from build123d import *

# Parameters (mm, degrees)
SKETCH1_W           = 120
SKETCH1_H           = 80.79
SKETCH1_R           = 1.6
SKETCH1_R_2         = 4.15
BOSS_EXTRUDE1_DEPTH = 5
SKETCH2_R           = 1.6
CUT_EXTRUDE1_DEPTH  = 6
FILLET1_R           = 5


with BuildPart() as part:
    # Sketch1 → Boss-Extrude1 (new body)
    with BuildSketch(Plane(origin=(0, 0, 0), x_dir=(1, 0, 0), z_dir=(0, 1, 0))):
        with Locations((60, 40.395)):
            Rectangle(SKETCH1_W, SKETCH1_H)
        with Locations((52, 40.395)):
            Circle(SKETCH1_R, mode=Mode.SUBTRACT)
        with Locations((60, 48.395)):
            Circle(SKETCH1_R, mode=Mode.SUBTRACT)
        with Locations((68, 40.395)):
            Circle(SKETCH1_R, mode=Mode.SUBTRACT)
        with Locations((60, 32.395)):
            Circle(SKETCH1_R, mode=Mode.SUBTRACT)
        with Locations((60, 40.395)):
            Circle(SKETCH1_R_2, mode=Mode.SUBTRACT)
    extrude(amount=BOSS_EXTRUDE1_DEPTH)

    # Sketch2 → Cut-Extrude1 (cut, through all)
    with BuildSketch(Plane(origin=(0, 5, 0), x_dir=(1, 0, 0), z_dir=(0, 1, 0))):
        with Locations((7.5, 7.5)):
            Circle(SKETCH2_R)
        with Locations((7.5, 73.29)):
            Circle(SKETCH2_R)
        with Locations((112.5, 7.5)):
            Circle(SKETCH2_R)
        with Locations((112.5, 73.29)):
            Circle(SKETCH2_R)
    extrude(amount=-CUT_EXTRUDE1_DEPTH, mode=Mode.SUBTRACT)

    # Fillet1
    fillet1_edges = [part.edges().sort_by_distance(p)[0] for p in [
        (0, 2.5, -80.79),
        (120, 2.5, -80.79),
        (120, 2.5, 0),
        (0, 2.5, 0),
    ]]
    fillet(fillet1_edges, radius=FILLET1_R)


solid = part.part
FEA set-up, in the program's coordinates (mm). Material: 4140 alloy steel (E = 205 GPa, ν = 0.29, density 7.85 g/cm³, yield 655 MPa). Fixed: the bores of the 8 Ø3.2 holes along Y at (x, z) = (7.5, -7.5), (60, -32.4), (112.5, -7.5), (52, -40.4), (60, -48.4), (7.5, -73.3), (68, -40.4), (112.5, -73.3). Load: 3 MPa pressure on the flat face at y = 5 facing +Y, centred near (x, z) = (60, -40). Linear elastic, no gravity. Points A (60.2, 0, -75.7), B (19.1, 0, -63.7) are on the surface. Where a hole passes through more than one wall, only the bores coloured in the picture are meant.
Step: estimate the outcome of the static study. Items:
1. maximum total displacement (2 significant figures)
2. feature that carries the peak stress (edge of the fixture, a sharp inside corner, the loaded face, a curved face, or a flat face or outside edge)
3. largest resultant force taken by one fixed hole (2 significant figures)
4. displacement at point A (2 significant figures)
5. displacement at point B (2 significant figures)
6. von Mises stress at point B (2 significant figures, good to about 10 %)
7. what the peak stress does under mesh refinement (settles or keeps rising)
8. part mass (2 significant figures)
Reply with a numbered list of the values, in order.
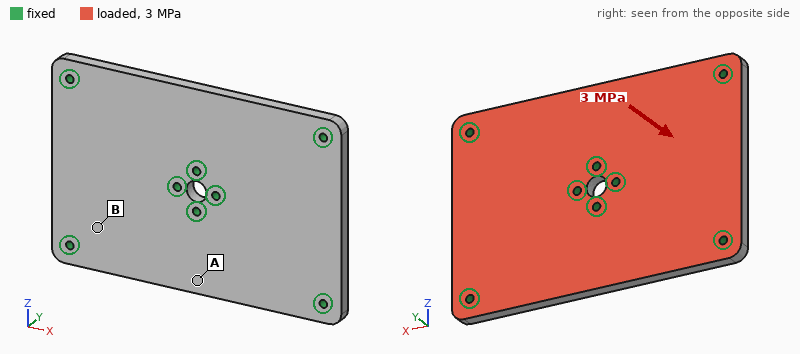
1. 0.15 mm
2. edge of the fixture
3. 4.0 kN
4. 0.12 mm
5. 0.044 mm
6. 130 MPa
7. keeps rising
8. 380 g
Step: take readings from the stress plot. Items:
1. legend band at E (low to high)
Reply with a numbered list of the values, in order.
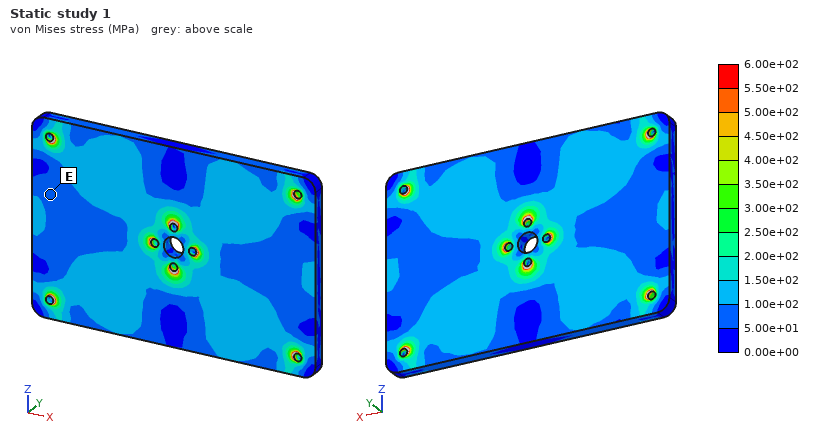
1. 5.00e+01 to 1.00e+02 MPa
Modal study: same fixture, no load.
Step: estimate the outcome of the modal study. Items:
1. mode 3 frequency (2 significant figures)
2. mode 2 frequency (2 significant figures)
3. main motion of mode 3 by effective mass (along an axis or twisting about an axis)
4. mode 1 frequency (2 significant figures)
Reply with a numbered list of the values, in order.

1. 5900 Hz
2. 4600 Hz
3. twisting about Z
4. 4500 Hz
